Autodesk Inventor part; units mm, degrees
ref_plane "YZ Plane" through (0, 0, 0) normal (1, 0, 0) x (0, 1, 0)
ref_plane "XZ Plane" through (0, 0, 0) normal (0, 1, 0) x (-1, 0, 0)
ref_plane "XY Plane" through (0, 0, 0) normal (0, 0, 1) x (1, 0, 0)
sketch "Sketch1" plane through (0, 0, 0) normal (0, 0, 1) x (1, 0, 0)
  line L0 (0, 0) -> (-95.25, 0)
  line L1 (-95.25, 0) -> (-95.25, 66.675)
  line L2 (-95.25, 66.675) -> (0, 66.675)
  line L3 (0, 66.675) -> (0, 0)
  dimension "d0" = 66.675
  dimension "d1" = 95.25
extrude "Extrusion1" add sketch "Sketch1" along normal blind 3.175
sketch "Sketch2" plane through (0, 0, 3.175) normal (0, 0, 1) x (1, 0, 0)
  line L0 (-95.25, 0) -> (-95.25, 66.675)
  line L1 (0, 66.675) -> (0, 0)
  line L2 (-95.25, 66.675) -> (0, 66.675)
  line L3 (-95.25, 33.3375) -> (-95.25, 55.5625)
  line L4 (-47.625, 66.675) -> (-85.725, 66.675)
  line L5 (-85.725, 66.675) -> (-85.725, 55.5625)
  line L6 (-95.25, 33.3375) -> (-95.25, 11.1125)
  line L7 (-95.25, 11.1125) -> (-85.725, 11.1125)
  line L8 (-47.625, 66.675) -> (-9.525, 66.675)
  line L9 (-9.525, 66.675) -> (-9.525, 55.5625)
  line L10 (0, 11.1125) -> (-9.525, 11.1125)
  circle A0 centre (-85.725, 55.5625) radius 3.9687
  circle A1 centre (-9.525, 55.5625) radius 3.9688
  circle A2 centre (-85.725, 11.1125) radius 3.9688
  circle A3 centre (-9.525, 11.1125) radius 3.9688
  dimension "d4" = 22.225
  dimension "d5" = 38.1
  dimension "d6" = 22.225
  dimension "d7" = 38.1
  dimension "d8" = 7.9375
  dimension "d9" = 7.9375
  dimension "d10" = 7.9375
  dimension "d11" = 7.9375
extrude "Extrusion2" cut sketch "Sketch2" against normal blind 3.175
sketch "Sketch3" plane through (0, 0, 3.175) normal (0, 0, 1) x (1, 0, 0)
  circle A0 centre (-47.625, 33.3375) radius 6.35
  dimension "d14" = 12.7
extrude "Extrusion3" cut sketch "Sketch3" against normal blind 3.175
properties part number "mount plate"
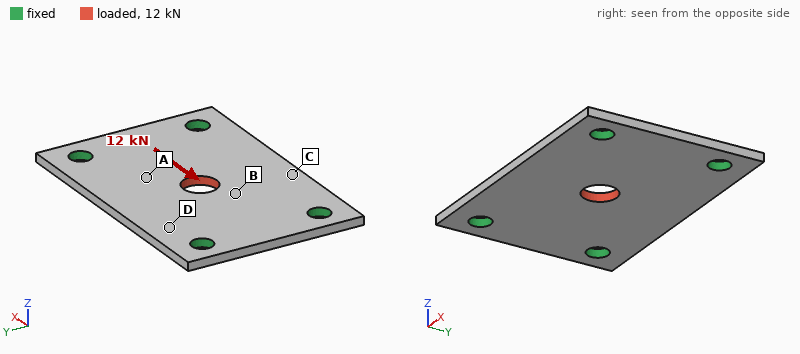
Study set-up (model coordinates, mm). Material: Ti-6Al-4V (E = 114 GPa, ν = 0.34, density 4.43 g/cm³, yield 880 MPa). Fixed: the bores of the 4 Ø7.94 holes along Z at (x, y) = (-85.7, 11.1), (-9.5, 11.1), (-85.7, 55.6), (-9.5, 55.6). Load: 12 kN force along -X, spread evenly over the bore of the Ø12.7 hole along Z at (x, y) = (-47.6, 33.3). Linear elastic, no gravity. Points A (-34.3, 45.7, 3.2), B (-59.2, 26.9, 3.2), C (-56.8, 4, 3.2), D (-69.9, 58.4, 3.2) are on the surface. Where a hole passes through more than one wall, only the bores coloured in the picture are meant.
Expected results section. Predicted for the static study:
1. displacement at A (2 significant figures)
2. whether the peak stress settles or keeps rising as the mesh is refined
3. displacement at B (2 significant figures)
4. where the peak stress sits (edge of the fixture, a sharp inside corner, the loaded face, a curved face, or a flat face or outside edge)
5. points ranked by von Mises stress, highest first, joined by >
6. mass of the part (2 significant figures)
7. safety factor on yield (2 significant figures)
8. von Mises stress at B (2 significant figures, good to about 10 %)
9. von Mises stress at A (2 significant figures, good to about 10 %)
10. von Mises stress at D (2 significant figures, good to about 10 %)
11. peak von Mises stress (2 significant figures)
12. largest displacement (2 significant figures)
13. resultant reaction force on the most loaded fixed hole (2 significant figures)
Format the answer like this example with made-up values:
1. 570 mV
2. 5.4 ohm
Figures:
1. 10 µm
2. settles
3. 14 µm
4. the loaded face
5. B > A > D > C
6. 85 g
7. 5.4
8. 68 MPa
9. 48 MPa
10. 27 MPa
11. 160 MPa
12. 20 µm
13. 3.2 kN
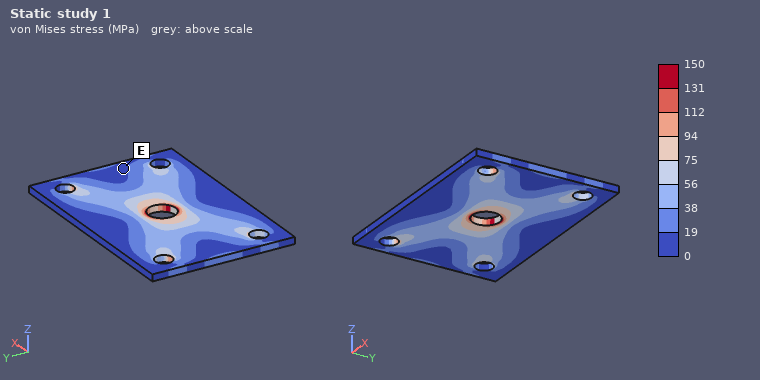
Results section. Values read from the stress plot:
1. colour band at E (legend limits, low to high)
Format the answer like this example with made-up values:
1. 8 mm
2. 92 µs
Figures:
1. 0 to 19 MPa
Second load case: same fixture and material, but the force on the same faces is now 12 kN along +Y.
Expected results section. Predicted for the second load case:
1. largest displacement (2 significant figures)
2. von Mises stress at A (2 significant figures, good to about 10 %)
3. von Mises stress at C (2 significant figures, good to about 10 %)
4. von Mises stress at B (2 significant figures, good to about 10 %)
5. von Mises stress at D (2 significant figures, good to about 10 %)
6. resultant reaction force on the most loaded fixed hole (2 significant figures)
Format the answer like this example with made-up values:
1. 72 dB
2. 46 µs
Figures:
1. 35 µm
2. 65 MPa
3. 36 MPa
4. 70 MPa
5. 39 MPa
6. 3.7 kN
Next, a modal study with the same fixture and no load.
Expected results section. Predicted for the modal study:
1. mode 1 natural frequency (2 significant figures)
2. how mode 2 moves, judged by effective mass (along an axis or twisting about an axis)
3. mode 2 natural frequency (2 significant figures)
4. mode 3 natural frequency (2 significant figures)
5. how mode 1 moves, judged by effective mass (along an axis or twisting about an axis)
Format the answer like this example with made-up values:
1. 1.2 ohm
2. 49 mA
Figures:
1. 3000 Hz
2. twisting about X
3. 3900 Hz
4. 6000 Hz
5. along Z
